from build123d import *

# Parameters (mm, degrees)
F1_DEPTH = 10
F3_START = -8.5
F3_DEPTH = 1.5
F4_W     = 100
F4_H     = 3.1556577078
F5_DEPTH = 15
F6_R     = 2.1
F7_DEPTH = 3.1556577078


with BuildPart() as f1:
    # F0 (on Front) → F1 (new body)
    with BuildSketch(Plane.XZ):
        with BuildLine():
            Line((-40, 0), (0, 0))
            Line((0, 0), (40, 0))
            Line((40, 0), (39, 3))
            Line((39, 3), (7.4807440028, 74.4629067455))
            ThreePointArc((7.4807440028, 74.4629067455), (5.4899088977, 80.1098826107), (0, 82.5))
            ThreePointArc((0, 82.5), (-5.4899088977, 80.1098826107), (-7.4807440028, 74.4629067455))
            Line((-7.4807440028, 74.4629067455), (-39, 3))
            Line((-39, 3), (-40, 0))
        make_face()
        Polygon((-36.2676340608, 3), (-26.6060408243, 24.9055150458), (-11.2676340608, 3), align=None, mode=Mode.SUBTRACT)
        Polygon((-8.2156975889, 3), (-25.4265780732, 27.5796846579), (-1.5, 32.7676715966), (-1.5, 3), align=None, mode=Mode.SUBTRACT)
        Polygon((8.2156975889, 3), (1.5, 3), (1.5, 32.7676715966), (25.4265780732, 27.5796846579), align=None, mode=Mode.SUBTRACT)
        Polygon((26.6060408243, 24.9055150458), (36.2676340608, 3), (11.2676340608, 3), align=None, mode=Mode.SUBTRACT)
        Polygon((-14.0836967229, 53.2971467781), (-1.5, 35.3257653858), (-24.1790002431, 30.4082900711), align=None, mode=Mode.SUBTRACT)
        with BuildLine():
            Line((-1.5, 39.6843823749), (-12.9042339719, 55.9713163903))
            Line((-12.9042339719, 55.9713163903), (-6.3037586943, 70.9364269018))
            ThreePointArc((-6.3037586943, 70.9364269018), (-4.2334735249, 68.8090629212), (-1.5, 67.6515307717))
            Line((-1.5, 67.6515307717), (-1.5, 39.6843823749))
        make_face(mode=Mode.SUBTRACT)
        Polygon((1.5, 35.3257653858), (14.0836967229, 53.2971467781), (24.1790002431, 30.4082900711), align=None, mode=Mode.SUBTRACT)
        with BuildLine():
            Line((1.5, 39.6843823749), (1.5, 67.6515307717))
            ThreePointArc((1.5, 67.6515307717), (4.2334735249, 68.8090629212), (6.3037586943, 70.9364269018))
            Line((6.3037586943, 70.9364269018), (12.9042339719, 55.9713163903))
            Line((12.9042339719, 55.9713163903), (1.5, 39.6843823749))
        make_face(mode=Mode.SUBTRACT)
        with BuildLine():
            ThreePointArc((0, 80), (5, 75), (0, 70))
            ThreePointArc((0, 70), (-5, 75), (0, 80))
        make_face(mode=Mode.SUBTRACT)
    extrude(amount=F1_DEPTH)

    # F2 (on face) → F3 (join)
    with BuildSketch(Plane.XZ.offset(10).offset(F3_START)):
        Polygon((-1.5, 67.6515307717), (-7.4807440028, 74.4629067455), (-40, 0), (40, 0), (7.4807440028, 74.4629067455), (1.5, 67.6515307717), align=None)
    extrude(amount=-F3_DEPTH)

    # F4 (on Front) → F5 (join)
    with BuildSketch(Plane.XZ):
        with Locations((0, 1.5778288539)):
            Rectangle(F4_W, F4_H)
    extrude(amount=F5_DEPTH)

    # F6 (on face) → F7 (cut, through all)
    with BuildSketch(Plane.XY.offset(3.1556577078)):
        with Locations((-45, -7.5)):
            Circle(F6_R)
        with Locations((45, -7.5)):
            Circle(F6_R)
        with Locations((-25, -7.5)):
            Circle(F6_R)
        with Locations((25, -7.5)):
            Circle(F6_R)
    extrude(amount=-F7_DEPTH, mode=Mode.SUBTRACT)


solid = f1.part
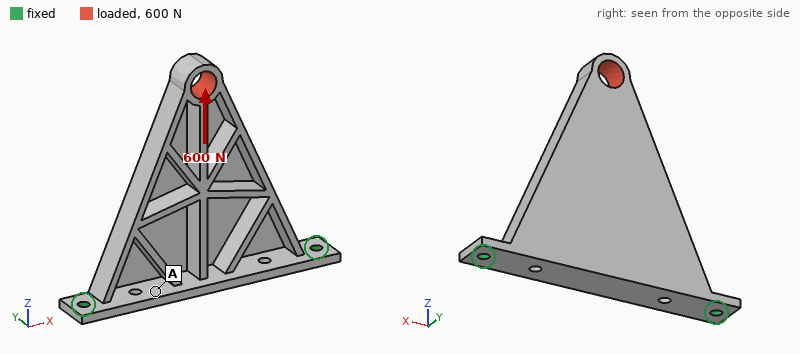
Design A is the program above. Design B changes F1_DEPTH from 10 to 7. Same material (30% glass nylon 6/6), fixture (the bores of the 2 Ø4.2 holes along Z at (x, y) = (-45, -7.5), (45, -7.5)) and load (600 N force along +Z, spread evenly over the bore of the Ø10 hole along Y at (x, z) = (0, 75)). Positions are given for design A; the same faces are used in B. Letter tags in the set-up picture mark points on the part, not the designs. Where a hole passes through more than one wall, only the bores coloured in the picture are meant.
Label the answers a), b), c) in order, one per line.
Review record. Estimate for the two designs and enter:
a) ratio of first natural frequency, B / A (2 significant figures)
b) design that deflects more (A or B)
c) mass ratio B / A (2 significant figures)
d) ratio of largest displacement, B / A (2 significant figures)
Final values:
a) 0.88
b) B
c) 0.83
d) 1.5
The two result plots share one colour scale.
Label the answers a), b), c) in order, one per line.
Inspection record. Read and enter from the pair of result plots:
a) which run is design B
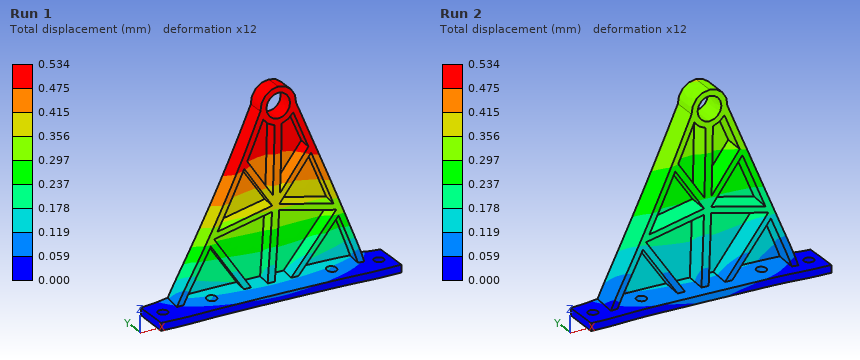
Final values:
a) Run 1
